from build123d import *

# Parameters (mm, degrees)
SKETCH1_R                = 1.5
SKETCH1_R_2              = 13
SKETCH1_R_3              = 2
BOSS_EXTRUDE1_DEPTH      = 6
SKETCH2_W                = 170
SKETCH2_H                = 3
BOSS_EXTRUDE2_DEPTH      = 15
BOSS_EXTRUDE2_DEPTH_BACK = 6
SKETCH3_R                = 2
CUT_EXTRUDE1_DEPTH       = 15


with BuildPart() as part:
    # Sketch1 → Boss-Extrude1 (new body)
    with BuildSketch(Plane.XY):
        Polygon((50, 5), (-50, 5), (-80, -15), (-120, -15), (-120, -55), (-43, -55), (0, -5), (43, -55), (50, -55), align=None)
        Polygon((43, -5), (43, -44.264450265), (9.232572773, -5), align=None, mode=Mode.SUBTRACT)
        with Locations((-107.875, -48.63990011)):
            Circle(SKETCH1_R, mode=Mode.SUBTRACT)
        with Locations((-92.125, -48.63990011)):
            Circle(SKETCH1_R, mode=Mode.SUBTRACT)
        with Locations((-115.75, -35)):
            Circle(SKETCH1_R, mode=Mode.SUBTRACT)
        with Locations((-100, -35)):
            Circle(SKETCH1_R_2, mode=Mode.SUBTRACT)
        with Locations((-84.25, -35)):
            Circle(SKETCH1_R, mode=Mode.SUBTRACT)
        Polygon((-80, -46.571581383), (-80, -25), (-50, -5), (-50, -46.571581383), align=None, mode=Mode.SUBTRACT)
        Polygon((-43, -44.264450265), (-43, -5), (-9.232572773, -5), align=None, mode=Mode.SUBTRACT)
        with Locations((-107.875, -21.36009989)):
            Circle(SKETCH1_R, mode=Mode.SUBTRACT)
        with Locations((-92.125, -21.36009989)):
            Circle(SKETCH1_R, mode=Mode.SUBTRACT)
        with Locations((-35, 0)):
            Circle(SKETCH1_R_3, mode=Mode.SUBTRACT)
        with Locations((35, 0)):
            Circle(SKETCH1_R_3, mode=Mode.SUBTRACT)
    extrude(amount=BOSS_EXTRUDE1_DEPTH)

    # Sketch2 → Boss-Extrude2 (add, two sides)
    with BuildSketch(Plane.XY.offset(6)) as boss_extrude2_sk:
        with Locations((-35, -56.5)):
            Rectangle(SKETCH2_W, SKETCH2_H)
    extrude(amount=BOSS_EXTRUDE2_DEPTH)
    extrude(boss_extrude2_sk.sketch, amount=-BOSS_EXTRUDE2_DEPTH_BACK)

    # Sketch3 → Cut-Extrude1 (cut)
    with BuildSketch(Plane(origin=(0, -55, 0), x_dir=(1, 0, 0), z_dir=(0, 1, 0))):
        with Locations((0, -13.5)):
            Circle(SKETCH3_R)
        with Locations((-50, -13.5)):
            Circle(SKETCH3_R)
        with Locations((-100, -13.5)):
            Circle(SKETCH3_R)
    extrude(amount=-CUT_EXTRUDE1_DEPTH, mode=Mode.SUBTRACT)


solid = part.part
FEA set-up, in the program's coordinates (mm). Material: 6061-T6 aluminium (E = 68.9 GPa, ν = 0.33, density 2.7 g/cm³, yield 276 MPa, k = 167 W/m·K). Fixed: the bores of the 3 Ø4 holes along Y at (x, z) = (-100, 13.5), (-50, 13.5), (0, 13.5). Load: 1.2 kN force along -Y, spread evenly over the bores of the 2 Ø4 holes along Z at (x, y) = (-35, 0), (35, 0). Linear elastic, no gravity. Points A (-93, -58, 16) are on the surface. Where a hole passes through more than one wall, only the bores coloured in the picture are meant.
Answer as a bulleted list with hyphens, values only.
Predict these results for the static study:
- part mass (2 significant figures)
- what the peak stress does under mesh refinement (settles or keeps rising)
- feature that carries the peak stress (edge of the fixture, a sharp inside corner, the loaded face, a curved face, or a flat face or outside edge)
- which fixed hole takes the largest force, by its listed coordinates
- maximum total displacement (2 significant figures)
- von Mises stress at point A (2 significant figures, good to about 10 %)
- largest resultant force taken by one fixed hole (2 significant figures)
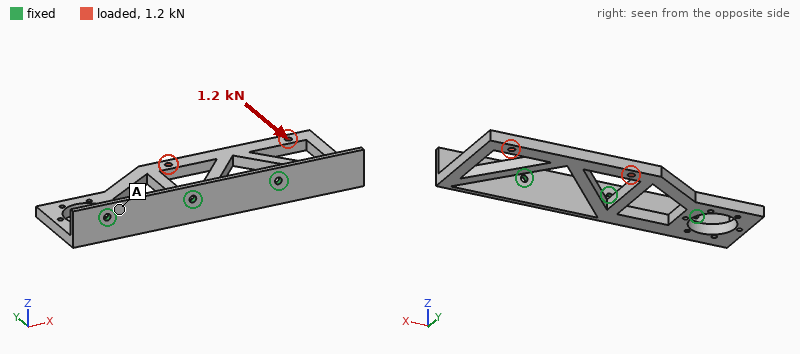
- 95 g
- keeps rising
- edge of the fixture
- (-50, 13.5)
- 0.93 mm
- 26 MPa
- 1.9 kN
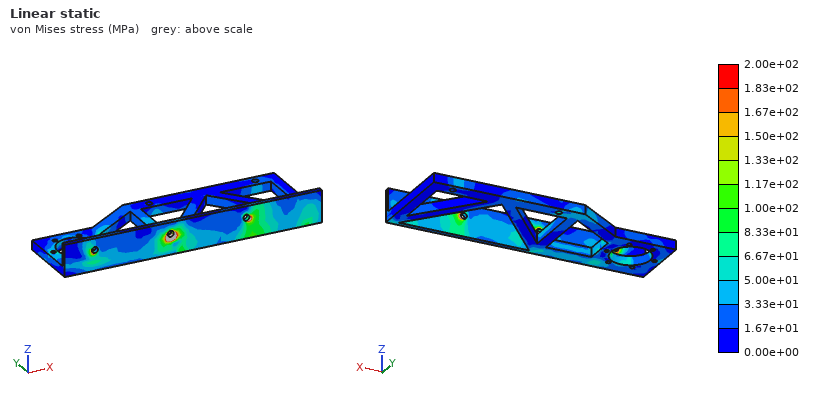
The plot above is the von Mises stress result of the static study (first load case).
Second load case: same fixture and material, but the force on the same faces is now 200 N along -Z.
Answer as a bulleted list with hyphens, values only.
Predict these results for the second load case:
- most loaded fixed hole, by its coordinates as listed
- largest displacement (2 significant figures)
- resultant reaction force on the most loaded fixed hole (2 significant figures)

- (0, 13.5)
- 1.7 mm
- 150 N
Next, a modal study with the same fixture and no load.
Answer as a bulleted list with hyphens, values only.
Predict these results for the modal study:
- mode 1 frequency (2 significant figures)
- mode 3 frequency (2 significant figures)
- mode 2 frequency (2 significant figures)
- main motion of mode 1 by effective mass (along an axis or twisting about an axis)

- 400 Hz
- 1100 Hz
- 1000 Hz
- along Z
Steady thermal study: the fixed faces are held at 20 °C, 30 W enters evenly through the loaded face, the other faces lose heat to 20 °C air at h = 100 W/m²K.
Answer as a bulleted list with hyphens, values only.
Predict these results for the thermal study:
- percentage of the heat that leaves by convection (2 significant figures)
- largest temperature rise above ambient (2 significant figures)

- 78 %
- 44 K
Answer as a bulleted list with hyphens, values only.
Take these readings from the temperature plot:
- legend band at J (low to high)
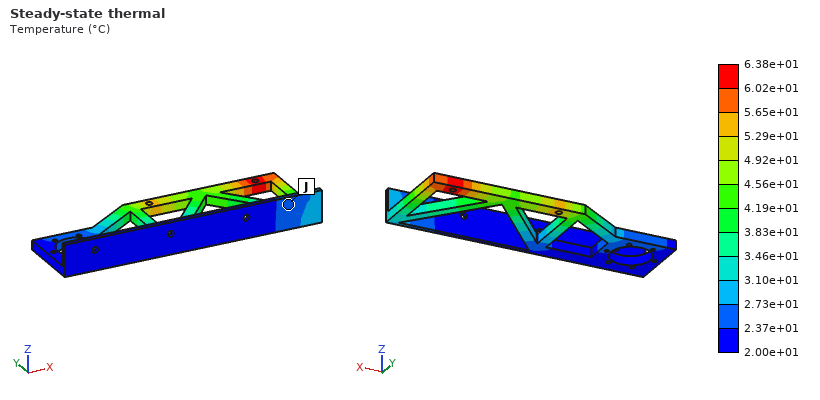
- 2.37e+01 to 2.73e+01 °C
